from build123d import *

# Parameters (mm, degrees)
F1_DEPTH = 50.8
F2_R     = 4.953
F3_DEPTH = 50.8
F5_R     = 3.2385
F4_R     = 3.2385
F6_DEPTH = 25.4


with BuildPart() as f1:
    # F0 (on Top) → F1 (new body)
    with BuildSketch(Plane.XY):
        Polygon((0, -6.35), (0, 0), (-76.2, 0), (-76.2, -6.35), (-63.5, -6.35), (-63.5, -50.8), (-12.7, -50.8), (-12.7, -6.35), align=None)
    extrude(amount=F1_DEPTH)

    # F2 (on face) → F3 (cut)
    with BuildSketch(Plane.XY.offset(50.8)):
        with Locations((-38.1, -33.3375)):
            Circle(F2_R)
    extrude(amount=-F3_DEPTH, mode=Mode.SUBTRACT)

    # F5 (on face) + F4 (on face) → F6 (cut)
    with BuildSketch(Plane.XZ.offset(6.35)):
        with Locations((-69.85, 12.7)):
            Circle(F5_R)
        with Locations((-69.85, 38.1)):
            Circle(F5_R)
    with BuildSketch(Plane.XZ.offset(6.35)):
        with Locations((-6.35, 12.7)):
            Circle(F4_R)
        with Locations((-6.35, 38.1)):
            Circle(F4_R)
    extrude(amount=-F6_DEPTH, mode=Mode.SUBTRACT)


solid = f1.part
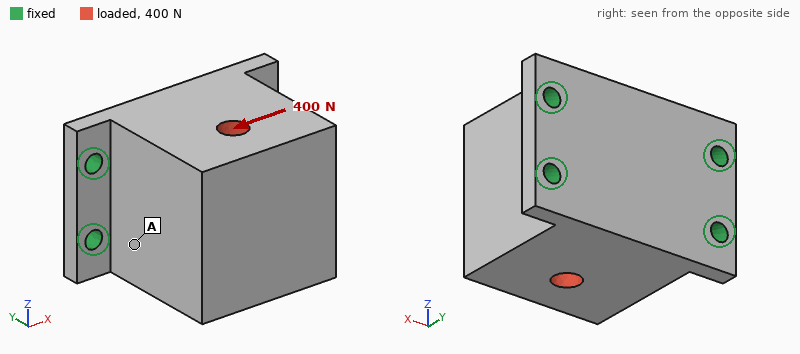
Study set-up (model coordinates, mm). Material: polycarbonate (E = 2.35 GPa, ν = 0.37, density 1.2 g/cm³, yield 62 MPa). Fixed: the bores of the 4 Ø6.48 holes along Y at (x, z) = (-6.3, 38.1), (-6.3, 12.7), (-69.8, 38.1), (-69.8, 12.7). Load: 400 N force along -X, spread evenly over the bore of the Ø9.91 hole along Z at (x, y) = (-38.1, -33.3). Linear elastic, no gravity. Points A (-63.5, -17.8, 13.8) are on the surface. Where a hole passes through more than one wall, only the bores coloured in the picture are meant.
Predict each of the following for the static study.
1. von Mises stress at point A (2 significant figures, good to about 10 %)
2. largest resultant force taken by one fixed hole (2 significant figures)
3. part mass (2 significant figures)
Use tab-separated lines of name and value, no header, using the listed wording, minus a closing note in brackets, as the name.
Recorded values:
von Mises stress at point A	0.39 MPa
largest resultant force taken by one fixed hole	150 N
part mass	160 g
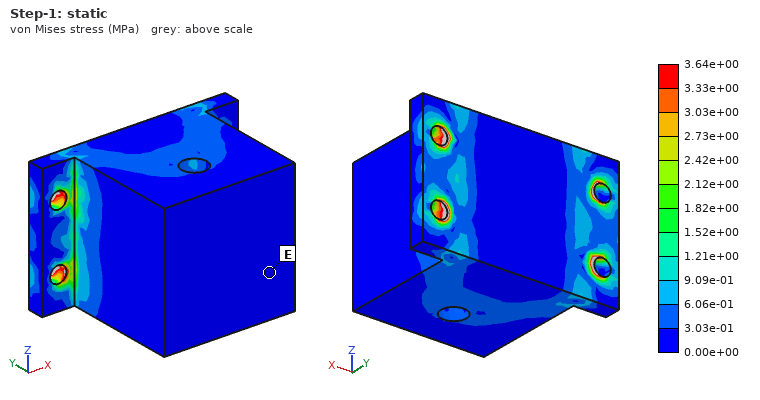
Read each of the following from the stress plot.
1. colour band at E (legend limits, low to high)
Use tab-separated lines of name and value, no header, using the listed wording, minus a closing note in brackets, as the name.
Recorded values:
colour band at E	0.00e+00 to 3.03e-01 MPa
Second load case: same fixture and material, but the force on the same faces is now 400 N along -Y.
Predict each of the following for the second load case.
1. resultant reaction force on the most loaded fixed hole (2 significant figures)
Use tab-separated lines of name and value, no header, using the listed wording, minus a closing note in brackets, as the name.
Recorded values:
resultant reaction force on the most loaded fixed hole	110 N
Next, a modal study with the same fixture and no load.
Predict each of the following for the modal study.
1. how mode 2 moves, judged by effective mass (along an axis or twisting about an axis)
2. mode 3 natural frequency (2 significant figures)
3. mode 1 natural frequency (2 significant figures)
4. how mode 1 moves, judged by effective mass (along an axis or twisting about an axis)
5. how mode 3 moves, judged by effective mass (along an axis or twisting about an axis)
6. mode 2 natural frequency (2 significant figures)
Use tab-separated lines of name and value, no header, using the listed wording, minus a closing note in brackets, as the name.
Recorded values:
how mode 2 moves, judged by effective mass	along X
mode 3 natural frequency	2100 Hz
mode 1 natural frequency	930 Hz
how mode 1 moves, judged by effective mass	along Z
how mode 3 moves, judged by effective mass	along Y
mode 2 natural frequency	1800 Hz
